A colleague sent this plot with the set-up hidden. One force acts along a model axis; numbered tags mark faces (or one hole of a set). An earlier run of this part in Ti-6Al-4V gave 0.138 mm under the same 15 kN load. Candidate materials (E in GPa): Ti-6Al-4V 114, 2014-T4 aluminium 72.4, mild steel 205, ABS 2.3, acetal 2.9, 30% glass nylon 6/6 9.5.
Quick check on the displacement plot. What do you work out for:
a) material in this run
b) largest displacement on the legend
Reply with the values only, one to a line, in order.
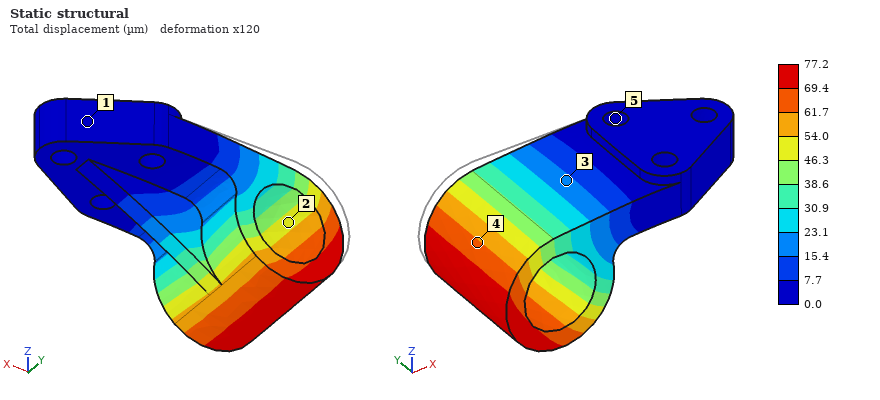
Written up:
mild steel
77.2 µm
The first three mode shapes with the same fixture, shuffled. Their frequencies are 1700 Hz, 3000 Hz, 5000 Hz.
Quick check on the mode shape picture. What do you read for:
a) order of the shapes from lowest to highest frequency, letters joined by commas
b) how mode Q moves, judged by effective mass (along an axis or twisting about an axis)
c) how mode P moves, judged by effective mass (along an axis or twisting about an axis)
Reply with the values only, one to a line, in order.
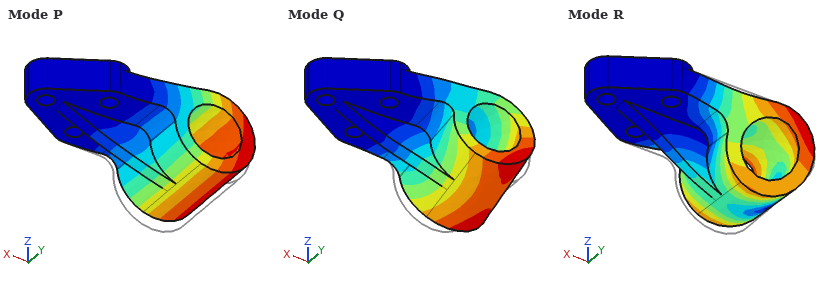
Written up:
P, Q, R
along Y
along Z
